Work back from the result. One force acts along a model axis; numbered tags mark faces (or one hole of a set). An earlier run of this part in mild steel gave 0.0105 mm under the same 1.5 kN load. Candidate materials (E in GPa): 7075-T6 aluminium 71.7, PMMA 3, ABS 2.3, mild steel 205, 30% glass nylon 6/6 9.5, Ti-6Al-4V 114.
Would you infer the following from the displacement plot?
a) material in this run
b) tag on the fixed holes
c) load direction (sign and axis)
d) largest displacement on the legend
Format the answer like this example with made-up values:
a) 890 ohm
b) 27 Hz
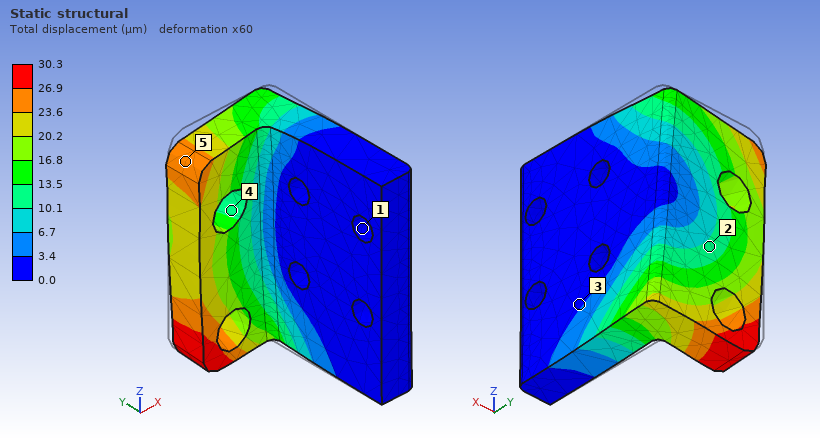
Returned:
a) 7075-T6 aluminium
b) 1
c) -Z
d) 30.3 µm
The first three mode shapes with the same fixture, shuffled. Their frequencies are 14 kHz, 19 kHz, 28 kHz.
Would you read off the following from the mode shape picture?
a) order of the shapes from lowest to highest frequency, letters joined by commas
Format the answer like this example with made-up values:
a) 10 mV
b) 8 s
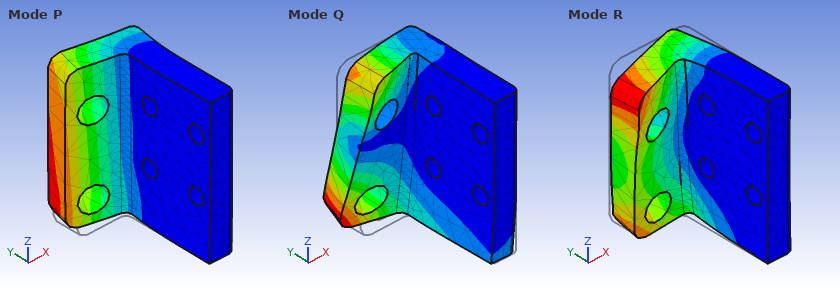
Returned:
a) P, R, Q
